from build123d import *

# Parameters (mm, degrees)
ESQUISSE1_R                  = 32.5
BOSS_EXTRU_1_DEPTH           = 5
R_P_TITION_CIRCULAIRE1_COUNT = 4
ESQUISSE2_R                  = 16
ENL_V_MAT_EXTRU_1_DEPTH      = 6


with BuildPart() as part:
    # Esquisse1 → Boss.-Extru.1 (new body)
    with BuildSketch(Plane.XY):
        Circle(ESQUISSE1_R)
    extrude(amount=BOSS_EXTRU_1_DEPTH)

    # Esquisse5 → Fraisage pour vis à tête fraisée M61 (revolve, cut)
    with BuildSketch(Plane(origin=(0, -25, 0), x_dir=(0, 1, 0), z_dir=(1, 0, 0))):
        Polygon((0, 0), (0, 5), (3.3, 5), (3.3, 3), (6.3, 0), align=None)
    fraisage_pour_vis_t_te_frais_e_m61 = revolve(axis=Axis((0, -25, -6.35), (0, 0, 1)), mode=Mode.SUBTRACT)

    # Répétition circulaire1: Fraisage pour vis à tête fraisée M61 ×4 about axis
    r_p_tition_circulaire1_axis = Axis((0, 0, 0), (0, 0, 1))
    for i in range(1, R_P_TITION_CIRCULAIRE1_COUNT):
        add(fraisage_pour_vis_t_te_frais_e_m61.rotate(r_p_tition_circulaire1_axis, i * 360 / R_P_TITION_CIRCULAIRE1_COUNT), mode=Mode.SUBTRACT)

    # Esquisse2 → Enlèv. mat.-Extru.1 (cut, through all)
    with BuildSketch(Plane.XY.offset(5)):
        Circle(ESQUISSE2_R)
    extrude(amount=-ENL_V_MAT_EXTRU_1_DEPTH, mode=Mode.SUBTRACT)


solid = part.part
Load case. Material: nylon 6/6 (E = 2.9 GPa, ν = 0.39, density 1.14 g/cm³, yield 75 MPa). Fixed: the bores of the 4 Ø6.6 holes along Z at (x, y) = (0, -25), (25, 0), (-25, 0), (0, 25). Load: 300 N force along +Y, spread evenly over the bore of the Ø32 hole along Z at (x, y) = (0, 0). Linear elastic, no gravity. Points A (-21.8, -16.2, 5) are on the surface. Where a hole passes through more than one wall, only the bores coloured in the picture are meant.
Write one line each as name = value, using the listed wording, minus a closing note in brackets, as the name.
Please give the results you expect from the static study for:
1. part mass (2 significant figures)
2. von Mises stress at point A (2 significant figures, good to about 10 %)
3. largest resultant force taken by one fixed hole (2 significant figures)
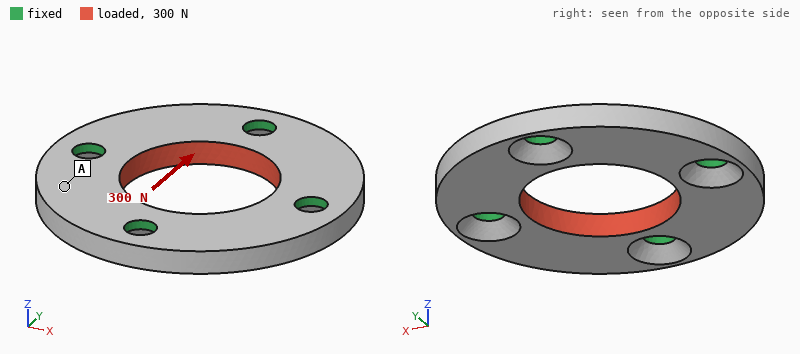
part mass = 13 g
von Mises stress at point A = 0.52 MPa
largest resultant force taken by one fixed hole = 76 N
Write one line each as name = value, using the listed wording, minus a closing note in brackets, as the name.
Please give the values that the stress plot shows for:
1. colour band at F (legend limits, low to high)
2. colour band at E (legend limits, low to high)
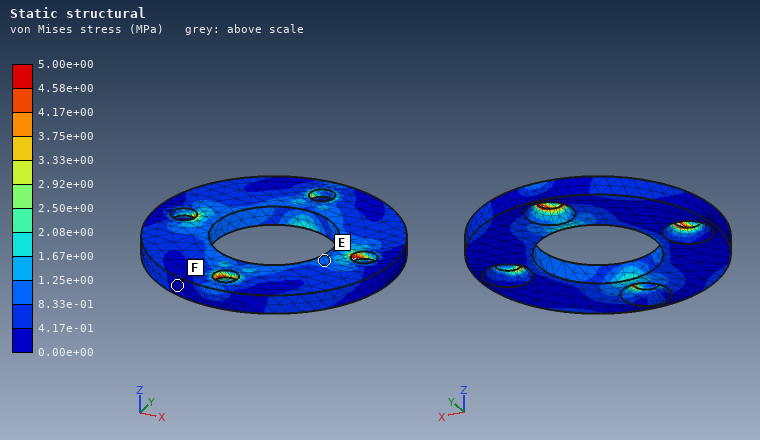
colour band at F = 0.00e+00 to 4.17e-01 MPa
colour band at E = 8.33e-01 to 1.25e+00 MPa
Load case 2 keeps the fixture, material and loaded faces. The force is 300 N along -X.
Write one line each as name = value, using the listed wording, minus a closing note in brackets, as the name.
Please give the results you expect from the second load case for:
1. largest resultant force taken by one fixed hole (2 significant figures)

largest resultant force taken by one fixed hole = 76 N
